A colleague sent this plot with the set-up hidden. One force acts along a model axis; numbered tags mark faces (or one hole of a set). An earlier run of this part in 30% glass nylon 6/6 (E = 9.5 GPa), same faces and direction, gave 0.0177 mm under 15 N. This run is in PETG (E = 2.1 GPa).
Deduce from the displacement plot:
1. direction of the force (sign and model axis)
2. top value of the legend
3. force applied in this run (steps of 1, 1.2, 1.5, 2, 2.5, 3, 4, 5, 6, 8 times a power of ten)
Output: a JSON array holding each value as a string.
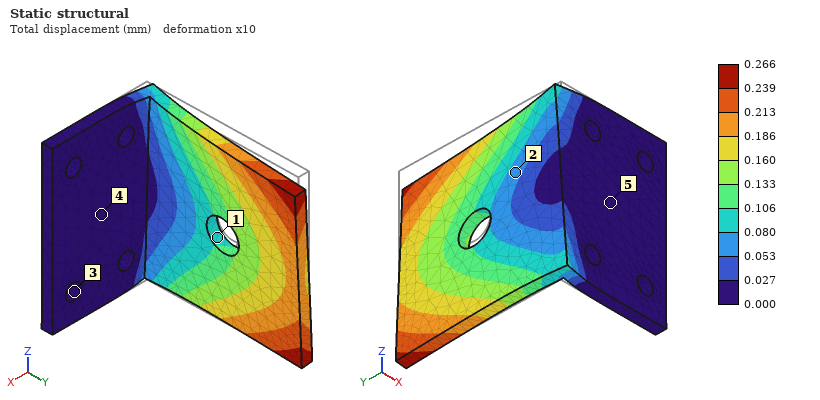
["-Z", "0.266 mm", "50 N"]
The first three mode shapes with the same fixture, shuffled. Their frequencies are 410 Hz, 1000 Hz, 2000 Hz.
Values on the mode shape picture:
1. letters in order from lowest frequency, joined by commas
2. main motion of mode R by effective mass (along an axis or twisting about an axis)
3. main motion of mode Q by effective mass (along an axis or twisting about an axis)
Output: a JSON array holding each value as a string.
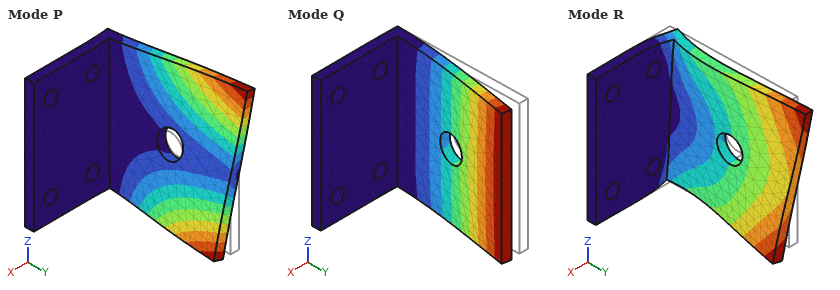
["Q, P, R", "along Z", "along X"]
